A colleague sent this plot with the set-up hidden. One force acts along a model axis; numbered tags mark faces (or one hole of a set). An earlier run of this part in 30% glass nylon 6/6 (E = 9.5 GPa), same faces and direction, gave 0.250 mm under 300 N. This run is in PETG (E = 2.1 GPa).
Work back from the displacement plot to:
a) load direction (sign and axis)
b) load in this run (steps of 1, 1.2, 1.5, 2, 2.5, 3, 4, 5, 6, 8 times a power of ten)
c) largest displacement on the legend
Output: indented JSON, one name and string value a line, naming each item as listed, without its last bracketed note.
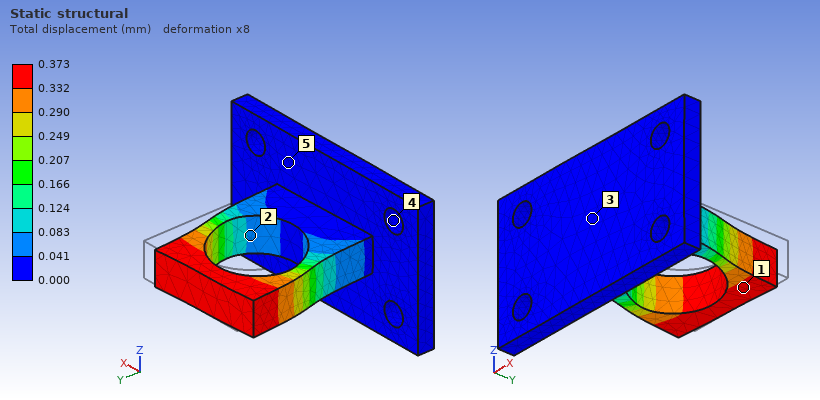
{
  "load direction": "-X",
  "load in this run": "100 N",
  "largest displacement on the legend": "0.373 mm"
}
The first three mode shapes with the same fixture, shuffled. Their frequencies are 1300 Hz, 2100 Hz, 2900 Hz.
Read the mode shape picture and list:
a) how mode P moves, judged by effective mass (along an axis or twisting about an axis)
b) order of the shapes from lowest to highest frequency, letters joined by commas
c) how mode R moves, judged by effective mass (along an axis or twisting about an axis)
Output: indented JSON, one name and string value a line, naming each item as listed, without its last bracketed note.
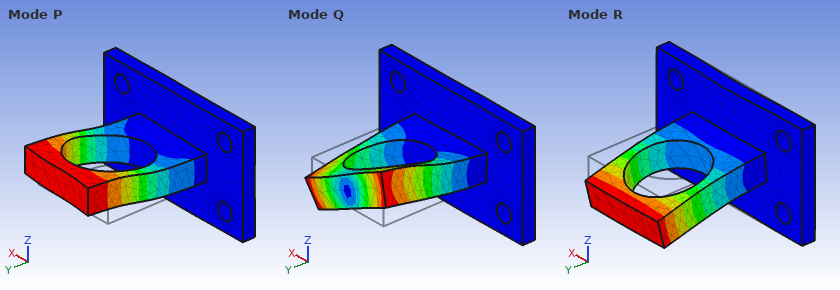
{
  "how mode P moves, judged by effective mass": "along X",
  "order of the shapes from lowest to highest frequency, letters joined by commas": "R, P, Q",
  "how mode R moves, judged by effective mass": "along Z"
}
